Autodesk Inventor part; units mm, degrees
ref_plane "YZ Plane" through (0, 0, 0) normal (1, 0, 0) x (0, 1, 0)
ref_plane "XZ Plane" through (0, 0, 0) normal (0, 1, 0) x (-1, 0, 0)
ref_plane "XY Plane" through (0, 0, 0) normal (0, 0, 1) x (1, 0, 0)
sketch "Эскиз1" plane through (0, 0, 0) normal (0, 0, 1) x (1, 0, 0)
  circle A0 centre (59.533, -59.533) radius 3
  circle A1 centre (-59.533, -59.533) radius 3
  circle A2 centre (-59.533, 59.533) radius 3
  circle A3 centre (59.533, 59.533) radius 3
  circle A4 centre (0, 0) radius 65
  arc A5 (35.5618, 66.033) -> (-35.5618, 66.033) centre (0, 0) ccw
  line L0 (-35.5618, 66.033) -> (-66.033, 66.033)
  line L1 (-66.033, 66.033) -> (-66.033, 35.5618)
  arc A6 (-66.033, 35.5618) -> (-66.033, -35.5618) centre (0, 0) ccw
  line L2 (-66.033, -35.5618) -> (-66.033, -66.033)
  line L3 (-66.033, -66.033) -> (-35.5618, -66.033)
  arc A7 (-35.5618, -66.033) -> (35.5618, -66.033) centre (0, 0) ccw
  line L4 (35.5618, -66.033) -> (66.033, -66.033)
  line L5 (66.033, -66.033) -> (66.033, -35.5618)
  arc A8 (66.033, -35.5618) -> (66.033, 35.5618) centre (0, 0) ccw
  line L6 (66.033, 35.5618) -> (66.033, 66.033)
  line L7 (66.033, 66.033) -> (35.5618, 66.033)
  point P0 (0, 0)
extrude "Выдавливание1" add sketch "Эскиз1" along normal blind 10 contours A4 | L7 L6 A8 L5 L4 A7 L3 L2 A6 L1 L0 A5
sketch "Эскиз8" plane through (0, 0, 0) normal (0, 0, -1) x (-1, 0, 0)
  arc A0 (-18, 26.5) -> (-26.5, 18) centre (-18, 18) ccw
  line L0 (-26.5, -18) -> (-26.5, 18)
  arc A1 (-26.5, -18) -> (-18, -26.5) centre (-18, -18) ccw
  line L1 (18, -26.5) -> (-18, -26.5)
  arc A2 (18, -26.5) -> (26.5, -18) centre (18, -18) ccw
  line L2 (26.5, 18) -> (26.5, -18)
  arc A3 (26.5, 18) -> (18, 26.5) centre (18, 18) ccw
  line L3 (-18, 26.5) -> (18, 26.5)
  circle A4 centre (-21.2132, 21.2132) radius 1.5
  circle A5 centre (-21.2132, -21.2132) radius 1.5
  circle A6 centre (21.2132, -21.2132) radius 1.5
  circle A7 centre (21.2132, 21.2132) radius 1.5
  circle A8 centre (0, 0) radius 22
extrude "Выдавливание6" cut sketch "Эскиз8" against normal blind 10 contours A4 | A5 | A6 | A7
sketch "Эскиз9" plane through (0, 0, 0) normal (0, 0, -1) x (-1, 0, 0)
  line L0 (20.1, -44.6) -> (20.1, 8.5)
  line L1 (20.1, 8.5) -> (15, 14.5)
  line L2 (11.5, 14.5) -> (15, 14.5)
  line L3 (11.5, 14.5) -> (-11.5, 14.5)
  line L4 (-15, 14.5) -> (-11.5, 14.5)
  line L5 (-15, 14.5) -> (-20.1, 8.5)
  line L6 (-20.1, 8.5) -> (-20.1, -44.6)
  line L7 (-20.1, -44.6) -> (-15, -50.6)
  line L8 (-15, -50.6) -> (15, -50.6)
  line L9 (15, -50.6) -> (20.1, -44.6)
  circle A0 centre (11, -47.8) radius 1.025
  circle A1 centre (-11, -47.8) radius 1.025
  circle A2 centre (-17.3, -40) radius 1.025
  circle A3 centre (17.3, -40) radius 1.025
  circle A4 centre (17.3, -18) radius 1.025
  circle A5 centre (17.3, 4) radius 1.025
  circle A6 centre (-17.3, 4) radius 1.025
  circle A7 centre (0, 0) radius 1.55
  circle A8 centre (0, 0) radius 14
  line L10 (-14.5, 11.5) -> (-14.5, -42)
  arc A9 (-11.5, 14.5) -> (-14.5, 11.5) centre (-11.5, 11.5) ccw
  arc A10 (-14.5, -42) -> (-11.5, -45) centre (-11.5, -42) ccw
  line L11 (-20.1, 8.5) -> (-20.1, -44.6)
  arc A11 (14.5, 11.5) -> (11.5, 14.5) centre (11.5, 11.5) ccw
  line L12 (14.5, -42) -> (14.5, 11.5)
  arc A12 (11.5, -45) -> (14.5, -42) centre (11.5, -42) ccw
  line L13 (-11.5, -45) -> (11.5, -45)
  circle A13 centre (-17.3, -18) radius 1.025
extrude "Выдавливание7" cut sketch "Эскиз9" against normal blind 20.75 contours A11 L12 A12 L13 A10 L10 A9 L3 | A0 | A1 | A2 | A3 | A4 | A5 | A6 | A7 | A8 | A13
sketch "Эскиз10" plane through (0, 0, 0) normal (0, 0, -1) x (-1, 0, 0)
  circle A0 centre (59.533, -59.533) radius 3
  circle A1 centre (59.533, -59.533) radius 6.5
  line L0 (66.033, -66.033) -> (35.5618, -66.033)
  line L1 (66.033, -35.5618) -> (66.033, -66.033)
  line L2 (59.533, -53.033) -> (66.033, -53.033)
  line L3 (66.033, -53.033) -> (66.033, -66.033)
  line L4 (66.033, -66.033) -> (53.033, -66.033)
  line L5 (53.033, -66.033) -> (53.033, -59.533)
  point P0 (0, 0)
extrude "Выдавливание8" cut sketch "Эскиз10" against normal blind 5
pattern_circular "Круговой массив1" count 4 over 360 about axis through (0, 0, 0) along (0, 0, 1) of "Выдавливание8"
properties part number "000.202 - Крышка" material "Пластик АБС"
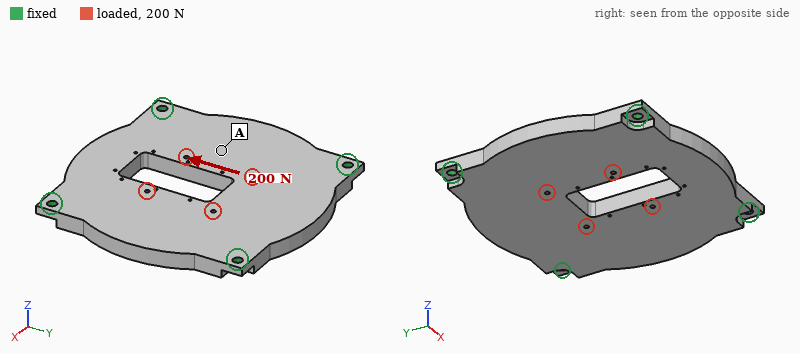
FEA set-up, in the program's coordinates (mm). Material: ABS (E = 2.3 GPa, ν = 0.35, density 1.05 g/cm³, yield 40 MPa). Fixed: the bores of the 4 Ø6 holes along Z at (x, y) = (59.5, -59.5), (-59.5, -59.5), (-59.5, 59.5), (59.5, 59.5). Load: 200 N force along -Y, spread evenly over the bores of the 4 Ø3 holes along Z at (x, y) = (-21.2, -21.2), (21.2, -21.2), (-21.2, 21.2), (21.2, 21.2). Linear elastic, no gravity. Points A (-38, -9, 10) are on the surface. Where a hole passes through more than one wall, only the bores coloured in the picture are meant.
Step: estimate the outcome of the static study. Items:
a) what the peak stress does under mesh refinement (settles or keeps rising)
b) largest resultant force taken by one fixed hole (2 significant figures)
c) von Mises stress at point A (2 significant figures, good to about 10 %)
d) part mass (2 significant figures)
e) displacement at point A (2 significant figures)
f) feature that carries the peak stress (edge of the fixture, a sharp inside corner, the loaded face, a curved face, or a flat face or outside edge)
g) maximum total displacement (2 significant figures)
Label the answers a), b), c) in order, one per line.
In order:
a) keeps rising
b) 54 N
c) 0.15 MPa
d) 180 g
e) 6.7 µm
f) edge of the fixture
g) 9.6 µm
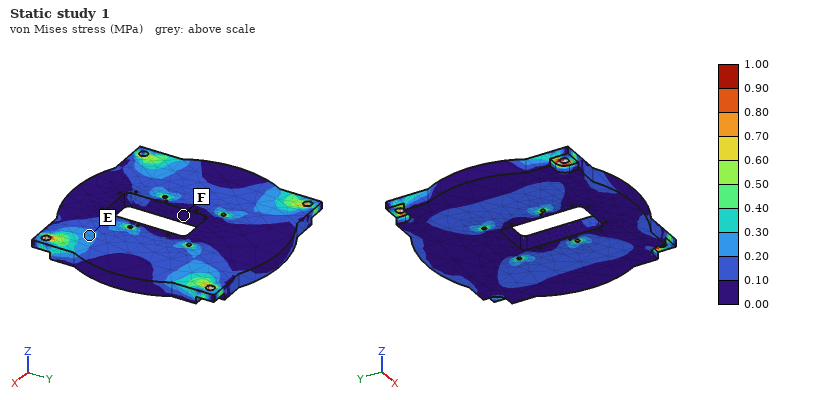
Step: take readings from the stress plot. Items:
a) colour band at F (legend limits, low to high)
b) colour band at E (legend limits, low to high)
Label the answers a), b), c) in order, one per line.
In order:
a) 0.00 to 0.10 MPa
b) 0.20 to 0.30 MPa
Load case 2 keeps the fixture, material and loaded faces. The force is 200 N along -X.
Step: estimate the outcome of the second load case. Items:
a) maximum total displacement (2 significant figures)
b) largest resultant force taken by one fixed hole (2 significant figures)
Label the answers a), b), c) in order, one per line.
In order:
a) 11 µm
b) 62 N
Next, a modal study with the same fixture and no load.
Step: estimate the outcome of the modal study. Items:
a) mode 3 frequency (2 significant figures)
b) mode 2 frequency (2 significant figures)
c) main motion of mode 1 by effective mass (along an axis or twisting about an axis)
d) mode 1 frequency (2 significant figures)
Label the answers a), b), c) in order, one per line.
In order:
a) 820 Hz
b) 810 Hz
c) along Z
d) 510 Hz
